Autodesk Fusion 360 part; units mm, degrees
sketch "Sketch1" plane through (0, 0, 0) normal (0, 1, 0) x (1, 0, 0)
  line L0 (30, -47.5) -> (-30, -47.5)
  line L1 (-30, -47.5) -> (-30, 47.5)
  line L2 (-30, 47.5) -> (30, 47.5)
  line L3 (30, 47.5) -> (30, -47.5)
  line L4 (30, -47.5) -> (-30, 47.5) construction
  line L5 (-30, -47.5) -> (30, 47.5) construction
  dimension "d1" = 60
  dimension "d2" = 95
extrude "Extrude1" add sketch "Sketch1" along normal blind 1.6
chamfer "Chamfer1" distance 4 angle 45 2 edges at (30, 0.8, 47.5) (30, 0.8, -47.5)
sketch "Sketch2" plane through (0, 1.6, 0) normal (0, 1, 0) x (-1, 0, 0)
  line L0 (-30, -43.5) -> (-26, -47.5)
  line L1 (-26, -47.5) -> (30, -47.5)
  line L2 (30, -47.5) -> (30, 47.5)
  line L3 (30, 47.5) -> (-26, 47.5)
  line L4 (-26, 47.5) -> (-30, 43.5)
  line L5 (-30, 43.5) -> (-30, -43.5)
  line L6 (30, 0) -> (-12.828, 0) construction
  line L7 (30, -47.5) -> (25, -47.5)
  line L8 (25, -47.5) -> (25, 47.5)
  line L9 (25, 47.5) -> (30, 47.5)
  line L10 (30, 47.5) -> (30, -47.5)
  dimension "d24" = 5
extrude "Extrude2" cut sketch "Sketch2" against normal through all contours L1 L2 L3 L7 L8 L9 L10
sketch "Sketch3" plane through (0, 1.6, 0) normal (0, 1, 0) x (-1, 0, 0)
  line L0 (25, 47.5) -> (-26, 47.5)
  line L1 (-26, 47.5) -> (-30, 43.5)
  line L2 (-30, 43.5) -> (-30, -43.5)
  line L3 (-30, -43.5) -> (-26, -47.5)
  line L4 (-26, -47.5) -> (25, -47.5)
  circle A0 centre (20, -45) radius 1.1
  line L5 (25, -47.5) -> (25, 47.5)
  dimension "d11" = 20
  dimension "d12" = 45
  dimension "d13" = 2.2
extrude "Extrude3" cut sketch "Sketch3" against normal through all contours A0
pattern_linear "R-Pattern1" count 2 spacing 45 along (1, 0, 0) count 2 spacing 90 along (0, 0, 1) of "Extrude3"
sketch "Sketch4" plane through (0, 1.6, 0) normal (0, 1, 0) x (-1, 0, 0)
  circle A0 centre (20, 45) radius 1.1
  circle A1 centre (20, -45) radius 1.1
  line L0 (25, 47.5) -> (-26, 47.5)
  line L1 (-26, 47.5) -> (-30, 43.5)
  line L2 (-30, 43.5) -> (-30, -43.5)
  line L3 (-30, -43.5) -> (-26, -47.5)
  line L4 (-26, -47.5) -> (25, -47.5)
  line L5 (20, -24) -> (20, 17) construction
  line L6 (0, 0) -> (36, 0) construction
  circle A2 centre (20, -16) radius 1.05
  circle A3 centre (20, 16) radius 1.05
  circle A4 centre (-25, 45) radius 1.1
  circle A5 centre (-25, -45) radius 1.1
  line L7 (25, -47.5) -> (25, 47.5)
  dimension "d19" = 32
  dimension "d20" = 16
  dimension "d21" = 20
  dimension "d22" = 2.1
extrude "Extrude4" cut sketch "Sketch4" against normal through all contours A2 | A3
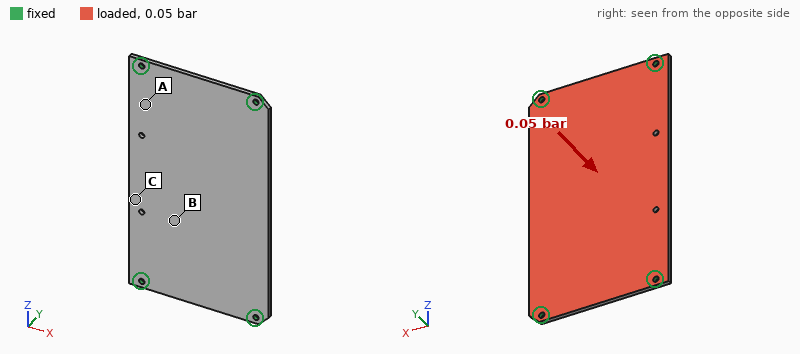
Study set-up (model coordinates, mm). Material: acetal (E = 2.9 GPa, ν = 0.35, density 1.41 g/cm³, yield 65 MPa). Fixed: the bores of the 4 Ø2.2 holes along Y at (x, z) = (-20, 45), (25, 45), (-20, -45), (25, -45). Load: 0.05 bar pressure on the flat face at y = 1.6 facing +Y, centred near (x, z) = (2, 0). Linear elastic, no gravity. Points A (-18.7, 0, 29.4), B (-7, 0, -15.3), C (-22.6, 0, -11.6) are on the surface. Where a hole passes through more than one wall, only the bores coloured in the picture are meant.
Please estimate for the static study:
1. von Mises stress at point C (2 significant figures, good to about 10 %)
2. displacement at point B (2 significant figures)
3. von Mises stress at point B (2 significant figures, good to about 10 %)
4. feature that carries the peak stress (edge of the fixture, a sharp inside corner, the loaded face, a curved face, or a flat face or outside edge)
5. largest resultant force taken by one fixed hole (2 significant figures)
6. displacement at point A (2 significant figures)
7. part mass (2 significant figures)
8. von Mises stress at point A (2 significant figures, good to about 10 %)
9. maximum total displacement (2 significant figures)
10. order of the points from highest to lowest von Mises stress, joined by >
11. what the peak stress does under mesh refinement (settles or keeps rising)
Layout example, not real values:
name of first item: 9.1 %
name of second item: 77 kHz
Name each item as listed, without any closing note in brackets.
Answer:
von Mises stress at point C: 4.4 MPa
displacement at point B: 0.99 mm
von Mises stress at point B: 3.2 MPa
feature that carries the peak stress: edge of the fixture
largest resultant force taken by one fixed hole: 6.5 N
displacement at point A: 0.45 mm
part mass: 12 g
von Mises stress at point A: 1.4 MPa
maximum total displacement: 1.2 mm
order of the points from highest to lowest von Mises stress, joined by >: C > B > A
what the peak stress does under mesh refinement: keeps rising
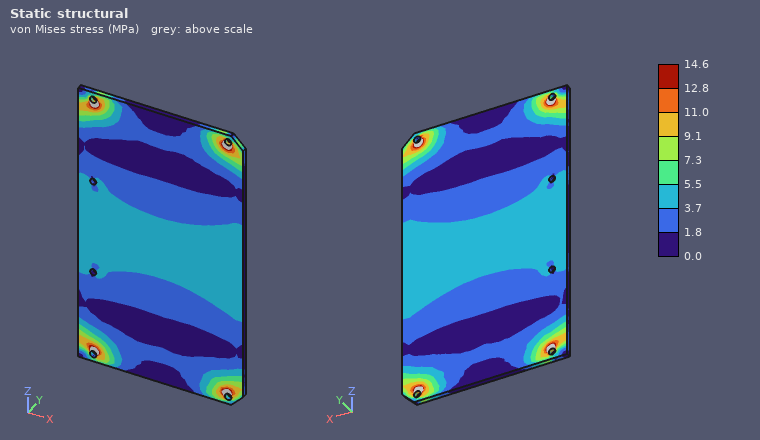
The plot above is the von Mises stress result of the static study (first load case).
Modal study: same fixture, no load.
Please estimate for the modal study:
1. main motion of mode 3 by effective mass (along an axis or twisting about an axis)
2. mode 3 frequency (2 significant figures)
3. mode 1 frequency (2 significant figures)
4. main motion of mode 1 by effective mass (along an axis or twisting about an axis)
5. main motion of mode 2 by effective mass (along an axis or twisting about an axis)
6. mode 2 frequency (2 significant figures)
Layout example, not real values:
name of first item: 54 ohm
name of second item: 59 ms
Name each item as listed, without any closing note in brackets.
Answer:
main motion of mode 3 by effective mass: twisting about X
mode 3 frequency: 680 Hz
mode 1 frequency: 240 Hz
main motion of mode 1 by effective mass: along Y
main motion of mode 2 by effective mass: twisting about Z
mode 2 frequency: 420 Hz
